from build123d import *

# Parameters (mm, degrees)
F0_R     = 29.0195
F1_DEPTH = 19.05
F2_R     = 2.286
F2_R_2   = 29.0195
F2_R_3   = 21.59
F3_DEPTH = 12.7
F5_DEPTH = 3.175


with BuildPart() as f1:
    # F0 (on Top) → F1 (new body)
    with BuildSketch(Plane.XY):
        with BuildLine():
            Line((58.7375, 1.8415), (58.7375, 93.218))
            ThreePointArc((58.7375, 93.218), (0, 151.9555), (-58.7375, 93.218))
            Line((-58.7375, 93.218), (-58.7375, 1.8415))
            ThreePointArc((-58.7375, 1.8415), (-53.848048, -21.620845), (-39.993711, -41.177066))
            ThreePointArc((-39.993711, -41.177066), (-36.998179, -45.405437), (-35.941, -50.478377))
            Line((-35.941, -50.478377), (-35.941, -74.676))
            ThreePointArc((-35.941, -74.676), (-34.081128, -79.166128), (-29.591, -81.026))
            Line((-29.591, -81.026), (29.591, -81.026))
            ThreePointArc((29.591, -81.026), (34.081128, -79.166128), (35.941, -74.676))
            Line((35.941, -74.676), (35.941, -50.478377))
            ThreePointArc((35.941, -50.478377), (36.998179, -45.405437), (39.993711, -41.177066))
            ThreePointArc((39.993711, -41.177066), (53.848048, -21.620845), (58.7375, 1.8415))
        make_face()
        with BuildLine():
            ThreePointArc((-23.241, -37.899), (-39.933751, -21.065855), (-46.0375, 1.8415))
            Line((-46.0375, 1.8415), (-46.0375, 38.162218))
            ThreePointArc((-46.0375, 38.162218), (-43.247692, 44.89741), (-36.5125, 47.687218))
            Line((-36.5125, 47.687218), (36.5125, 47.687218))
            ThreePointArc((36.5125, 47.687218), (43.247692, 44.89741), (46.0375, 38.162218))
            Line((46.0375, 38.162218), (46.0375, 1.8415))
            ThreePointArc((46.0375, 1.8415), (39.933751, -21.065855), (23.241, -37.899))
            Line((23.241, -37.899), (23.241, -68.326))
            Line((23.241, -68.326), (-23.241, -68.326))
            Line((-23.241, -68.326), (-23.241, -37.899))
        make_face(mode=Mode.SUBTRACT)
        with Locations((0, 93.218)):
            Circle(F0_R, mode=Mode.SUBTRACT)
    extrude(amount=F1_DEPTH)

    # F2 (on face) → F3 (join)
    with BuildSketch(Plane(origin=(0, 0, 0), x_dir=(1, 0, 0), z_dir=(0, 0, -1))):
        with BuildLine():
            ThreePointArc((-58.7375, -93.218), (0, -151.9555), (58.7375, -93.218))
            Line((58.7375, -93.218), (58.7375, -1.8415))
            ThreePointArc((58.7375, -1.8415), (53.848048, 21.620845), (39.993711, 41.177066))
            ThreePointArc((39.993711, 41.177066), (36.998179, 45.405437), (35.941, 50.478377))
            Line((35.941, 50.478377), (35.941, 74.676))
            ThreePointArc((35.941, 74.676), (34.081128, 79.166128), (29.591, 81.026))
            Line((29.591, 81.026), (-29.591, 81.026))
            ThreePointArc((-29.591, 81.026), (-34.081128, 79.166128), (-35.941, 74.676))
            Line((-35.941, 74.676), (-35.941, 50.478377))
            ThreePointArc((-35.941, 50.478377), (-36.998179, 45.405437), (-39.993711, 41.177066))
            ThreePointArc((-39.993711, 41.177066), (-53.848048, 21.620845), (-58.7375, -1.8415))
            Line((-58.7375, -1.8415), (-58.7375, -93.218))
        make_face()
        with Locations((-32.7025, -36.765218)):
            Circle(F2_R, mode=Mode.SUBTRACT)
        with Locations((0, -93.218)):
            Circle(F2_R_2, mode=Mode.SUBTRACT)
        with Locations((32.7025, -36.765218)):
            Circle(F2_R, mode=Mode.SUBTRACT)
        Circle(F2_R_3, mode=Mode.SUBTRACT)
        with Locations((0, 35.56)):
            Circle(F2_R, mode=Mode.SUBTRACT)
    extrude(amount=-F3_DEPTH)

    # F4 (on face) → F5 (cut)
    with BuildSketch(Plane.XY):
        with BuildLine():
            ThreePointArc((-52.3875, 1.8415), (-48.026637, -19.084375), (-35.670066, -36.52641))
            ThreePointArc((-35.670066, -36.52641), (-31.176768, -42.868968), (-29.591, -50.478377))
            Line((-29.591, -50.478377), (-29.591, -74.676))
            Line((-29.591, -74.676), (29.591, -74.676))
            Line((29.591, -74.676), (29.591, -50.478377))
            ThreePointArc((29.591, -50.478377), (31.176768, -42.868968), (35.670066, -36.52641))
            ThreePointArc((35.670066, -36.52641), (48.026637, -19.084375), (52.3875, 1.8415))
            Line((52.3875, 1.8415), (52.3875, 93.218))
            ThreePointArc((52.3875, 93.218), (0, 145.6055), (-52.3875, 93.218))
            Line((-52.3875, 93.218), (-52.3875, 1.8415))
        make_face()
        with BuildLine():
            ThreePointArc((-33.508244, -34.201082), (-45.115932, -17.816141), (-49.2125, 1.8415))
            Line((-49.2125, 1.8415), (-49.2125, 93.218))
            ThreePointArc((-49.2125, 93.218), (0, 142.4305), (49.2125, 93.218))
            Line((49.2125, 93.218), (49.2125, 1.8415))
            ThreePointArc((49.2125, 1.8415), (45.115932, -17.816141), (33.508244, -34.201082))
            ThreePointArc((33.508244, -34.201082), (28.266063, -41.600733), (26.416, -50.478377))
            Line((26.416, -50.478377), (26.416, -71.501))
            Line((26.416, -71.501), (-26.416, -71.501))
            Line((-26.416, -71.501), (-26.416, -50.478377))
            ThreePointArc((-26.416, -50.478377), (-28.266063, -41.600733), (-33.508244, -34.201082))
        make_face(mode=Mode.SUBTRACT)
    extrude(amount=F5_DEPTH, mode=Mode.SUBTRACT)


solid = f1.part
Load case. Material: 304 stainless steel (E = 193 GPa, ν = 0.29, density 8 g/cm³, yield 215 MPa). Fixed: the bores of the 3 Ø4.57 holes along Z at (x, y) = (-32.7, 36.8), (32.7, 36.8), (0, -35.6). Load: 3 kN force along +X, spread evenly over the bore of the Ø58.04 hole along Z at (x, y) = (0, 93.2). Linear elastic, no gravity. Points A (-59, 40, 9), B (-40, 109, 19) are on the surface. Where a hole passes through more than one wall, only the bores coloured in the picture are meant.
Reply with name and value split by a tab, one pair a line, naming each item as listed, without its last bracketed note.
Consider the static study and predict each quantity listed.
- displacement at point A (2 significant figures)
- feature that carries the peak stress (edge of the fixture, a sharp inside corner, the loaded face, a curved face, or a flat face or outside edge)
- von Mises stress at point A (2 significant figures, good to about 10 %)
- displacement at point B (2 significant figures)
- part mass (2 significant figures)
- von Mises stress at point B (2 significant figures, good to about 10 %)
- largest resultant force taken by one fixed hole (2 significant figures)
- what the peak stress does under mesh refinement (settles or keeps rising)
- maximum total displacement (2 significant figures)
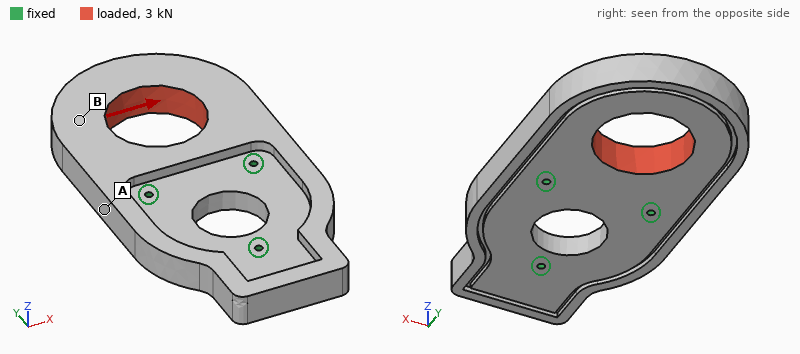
displacement at point A	1.5 µm
feature that carries the peak stress	edge of the fixture
von Mises stress at point A	5.5 MPa
displacement at point B	6.1 µm
part mass	2.5 kg
von Mises stress at point B	1.9 MPa
largest resultant force taken by one fixed hole	2.6 kN
what the peak stress does under mesh refinement	keeps rising
maximum total displacement	7.6 µm
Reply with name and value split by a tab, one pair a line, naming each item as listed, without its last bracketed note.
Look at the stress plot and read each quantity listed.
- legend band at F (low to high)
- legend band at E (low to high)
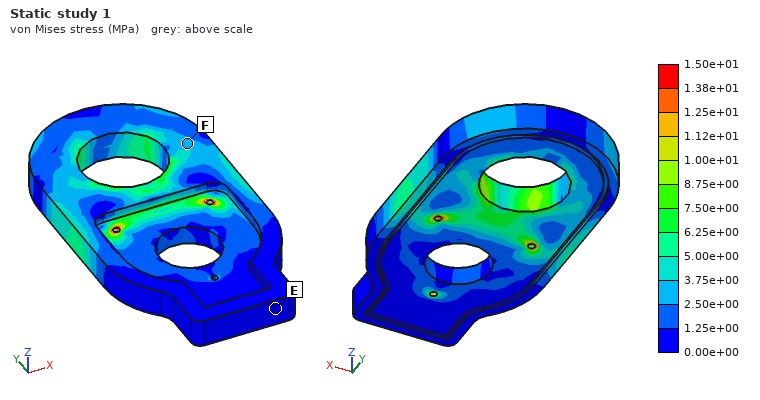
legend band at F	2.50e+00 to 3.75e+00 MPa
legend band at E	0.00e+00 to 1.25e+00 MPa
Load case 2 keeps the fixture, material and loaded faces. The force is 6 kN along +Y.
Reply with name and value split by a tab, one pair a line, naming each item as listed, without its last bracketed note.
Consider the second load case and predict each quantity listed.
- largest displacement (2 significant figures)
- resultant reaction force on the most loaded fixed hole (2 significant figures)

largest displacement	8.8 µm
resultant reaction force on the most loaded fixed hole	2.7 kN
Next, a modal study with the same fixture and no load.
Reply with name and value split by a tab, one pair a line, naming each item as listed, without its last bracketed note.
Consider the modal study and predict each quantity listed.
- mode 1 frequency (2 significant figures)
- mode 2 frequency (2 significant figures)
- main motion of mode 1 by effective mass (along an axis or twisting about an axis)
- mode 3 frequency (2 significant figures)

mode 1 frequency	880 Hz
mode 2 frequency	2300 Hz
main motion of mode 1 by effective mass	along Z
mode 3 frequency	3000 Hz
